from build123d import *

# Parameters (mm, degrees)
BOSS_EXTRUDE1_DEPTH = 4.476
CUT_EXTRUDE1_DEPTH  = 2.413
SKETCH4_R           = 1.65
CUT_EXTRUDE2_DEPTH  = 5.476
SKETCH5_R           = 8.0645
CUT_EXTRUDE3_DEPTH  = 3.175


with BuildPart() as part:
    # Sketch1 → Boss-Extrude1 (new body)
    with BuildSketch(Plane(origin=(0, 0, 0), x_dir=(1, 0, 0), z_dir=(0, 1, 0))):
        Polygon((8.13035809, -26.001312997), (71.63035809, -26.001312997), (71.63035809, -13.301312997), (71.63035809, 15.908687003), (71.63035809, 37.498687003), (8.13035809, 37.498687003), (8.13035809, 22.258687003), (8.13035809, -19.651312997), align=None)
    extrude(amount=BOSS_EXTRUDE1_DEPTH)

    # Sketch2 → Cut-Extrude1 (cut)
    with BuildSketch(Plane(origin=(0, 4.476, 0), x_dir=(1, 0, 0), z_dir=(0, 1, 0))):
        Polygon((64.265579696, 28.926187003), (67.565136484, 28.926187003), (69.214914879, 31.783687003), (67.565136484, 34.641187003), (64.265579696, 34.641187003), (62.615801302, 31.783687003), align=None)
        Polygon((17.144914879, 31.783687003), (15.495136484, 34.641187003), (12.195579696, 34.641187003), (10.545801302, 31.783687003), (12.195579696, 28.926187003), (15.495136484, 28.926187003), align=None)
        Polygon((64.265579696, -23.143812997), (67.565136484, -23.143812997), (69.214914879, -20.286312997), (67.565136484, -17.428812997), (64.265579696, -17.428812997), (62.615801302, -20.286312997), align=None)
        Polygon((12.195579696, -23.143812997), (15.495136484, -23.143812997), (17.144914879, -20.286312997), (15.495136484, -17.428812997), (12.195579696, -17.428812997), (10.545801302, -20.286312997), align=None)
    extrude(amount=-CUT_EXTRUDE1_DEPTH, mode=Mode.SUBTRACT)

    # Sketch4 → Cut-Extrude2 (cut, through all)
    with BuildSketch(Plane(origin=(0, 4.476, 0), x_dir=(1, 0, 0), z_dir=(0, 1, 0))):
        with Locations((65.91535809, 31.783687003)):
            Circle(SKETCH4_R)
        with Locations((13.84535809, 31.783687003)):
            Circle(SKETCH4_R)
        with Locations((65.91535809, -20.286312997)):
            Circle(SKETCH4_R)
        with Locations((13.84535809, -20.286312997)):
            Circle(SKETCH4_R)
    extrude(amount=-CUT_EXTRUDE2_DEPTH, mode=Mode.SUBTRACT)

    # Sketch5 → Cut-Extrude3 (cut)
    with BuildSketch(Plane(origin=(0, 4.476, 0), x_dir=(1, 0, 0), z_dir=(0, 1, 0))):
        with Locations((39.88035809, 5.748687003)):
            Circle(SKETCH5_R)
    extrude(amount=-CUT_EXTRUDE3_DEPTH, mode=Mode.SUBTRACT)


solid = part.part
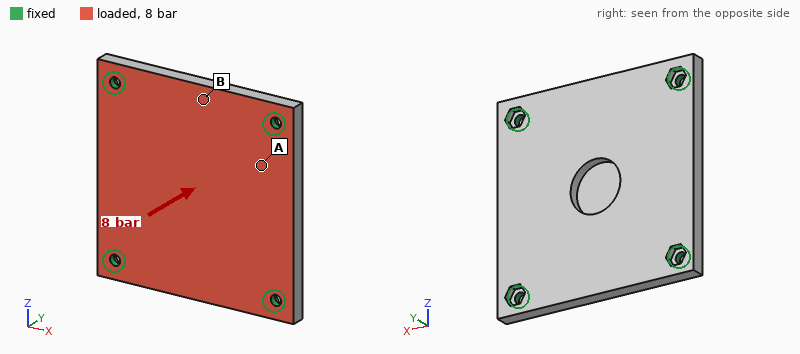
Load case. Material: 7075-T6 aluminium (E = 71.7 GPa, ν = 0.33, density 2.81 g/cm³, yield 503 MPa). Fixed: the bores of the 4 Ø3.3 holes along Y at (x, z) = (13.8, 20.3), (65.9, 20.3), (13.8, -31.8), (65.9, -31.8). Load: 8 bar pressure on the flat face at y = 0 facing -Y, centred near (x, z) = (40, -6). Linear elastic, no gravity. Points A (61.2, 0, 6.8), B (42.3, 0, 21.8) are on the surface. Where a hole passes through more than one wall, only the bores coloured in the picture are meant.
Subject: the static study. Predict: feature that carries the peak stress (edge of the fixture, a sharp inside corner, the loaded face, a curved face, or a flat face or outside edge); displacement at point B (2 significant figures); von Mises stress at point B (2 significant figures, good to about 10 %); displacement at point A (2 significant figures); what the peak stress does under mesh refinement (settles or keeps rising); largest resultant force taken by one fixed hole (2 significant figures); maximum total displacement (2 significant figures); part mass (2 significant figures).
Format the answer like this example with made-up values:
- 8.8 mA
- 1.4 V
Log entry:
- edge of the fixture
- 0.068 mm
- 41 MPa
- 0.064 mm
- keeps rising
- 1.2 kN
- 0.14 mm
- 48 g
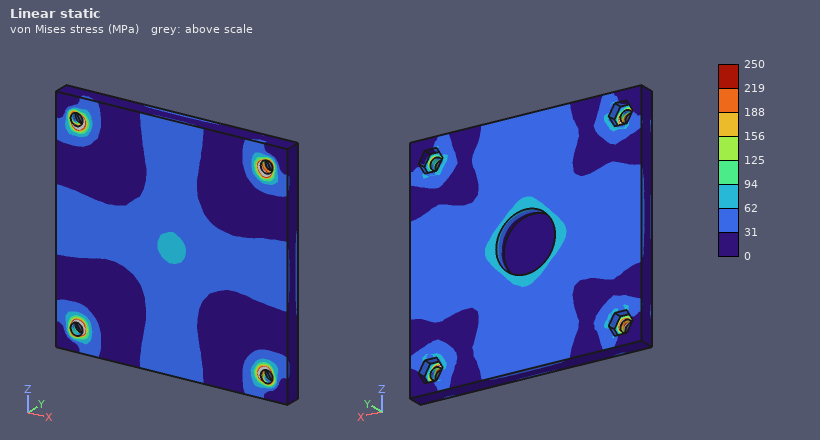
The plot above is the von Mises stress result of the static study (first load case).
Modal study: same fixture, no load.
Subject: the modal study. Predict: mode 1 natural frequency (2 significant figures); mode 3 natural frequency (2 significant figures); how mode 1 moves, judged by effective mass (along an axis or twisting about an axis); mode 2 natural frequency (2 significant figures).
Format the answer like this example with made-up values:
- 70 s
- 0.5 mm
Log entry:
- 4500 Hz
- 7400 Hz
- along Y
- 7400 Hz
